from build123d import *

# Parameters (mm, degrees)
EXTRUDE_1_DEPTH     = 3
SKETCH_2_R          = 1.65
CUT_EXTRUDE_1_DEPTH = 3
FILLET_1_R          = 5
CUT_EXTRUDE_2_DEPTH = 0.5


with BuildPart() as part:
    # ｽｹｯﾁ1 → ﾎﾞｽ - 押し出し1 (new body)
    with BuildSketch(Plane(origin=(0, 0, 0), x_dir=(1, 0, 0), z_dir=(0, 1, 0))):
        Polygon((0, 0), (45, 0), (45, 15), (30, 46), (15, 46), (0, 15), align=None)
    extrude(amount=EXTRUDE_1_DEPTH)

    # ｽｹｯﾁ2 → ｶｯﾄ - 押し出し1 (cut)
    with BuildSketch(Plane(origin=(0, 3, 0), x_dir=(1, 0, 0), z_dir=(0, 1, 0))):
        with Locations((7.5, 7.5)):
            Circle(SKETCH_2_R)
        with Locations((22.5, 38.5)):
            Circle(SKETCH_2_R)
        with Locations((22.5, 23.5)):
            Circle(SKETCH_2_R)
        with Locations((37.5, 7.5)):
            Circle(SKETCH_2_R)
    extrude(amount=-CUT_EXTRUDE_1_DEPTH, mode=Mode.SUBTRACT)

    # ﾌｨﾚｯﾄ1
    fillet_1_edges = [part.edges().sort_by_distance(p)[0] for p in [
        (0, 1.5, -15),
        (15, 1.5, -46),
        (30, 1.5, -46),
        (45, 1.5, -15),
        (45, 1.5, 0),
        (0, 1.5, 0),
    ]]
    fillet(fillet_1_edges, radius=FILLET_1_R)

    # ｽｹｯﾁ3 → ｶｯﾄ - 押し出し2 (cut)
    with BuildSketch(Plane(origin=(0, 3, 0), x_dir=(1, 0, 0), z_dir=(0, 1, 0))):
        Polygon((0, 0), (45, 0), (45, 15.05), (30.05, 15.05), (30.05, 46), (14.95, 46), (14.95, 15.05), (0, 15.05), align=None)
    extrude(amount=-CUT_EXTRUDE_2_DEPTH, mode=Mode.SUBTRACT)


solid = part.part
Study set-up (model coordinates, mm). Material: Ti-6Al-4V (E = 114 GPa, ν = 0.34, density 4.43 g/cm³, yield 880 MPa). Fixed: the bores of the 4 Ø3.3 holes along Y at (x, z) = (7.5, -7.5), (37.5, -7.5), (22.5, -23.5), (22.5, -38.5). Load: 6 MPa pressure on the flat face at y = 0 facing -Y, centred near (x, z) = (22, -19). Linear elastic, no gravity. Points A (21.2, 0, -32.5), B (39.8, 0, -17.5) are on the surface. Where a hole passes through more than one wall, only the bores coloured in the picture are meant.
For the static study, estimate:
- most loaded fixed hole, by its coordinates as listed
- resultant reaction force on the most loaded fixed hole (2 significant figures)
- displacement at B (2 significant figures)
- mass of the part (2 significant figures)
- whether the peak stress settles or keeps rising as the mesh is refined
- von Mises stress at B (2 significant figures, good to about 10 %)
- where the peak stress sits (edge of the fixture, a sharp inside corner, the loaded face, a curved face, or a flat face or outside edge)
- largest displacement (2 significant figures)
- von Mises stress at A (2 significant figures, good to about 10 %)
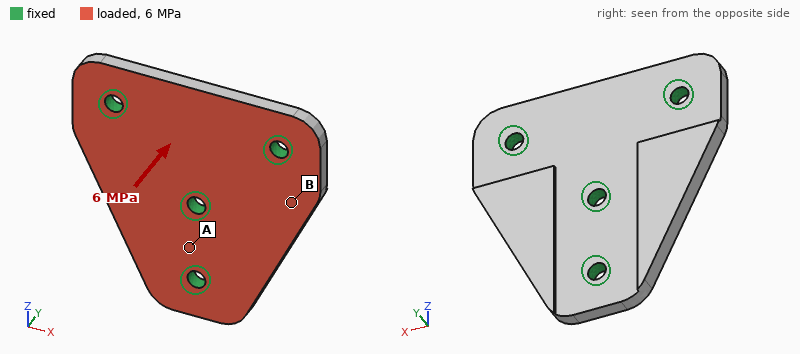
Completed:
(22.5, -23.5)
2.6 kN
0.069 mm
18 g
keeps rising
86 MPa
edge of the fixture
0.12 mm
220 MPa
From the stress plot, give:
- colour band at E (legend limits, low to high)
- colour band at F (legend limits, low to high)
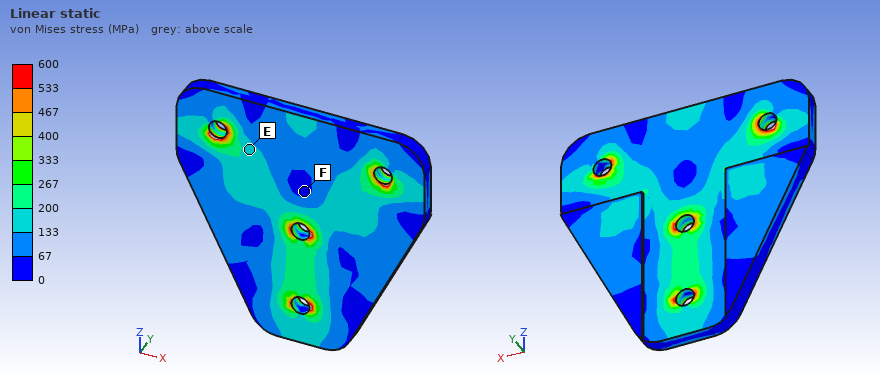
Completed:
133 to 200 MPa
0 to 67 MPa
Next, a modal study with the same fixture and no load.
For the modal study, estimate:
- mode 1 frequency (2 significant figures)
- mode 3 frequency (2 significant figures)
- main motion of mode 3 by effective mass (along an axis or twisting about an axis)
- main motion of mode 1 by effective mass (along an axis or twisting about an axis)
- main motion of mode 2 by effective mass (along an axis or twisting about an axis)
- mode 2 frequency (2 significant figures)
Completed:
12 kHz
16 kHz
along Y
twisting about Z
along Y
12 kHz
